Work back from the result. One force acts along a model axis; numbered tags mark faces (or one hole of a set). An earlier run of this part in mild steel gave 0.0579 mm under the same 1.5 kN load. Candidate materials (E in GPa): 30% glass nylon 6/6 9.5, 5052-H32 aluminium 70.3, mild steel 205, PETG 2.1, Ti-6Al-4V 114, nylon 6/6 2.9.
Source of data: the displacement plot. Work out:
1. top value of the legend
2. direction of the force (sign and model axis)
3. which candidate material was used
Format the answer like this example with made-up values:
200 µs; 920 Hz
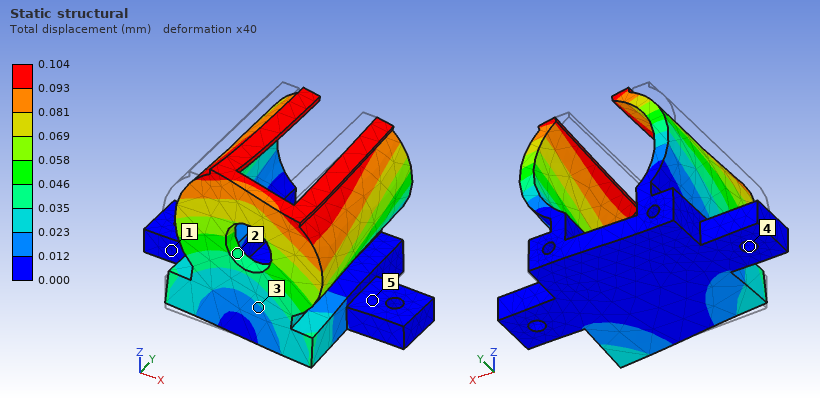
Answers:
0.104 mm; +X; Ti-6Al-4V
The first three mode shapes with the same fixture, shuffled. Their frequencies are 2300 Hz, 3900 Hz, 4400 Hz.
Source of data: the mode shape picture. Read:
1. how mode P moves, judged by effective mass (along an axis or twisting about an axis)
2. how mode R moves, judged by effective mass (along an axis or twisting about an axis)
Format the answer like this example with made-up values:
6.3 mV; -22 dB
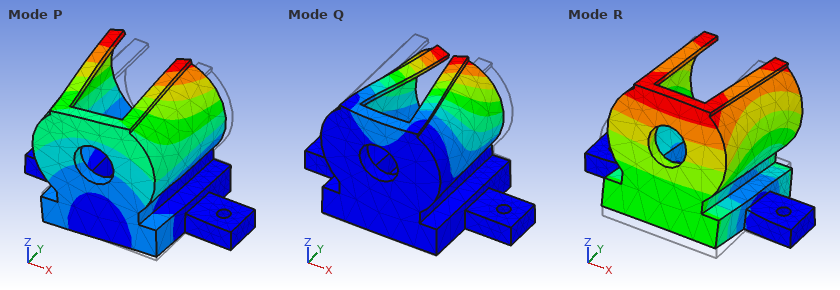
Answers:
along X; along Y
